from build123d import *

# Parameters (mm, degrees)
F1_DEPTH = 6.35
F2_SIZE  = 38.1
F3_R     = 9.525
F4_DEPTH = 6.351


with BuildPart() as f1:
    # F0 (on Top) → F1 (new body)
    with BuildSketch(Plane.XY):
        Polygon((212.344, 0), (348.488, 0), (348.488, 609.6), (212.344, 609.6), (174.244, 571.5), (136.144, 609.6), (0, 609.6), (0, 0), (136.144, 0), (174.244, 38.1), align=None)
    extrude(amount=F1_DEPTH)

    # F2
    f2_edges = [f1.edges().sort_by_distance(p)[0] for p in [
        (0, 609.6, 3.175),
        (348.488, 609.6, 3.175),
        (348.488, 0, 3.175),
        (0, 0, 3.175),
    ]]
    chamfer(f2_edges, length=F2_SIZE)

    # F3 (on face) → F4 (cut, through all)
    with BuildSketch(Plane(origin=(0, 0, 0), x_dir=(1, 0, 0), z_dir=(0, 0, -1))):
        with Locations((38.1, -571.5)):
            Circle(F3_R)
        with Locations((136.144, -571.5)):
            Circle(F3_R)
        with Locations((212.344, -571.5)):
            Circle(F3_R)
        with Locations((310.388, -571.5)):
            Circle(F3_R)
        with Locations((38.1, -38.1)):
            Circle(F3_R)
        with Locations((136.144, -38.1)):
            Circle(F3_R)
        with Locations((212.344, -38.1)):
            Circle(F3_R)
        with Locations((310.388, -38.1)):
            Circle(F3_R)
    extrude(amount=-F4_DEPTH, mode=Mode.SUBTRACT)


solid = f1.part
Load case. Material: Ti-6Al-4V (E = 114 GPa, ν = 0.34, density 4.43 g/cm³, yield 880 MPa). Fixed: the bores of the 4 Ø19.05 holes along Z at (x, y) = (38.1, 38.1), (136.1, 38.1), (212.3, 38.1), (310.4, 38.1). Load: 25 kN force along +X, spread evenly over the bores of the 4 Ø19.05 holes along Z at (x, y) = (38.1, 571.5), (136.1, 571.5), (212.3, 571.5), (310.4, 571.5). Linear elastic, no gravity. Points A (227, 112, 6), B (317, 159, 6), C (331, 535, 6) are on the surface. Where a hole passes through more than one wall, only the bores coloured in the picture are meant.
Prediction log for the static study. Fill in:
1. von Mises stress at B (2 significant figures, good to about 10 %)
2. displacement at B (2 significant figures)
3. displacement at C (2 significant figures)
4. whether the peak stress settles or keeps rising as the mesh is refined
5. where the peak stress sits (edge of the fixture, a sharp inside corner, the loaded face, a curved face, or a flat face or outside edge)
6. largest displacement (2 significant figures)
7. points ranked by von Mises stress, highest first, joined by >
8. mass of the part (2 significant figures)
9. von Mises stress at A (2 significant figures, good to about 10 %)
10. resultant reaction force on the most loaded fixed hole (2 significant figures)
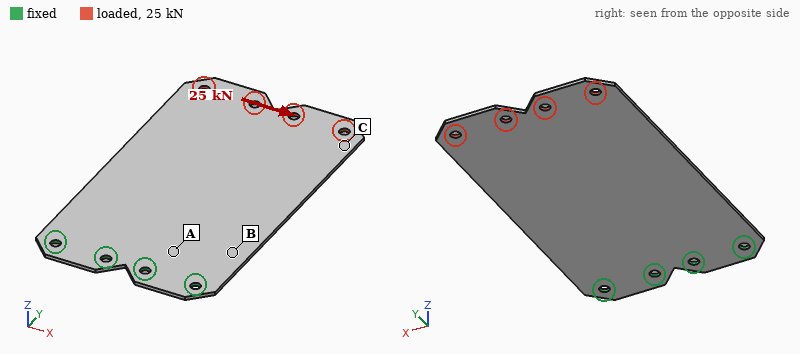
67 MPa
0.13 mm
0.69 mm
keeps rising
edge of the fixture
0.80 mm
B > A > C
5.7 kg
34 MPa
45 kN
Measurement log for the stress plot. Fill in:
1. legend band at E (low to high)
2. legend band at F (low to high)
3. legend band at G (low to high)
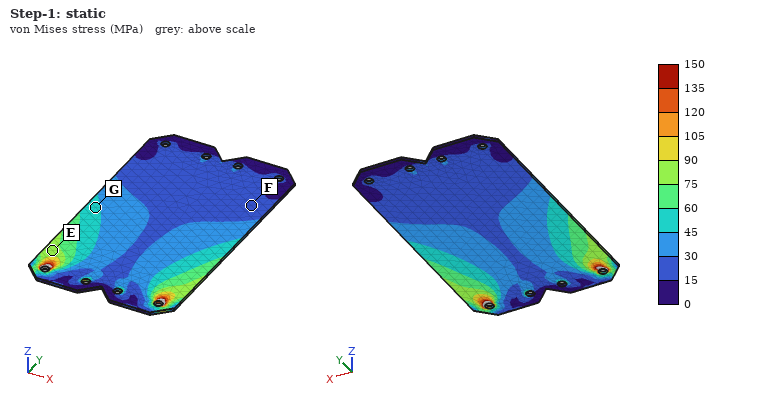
75 to 90 MPa
15 to 30 MPa
45 to 60 MPa
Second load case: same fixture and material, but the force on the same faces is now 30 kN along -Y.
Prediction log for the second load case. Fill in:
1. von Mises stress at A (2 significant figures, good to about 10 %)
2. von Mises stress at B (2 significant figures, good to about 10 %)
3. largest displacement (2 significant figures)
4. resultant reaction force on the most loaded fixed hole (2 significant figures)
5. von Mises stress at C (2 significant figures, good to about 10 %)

13 MPa
13 MPa
71 µm
8.0 kN
15 MPa
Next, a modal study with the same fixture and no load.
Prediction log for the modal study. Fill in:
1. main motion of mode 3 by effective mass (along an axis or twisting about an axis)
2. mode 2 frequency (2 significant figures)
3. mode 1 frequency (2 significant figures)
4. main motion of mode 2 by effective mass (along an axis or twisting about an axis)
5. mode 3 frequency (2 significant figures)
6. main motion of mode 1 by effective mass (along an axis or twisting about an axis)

along Z
61 Hz
17 Hz
twisting about Y
110 Hz
along Z
